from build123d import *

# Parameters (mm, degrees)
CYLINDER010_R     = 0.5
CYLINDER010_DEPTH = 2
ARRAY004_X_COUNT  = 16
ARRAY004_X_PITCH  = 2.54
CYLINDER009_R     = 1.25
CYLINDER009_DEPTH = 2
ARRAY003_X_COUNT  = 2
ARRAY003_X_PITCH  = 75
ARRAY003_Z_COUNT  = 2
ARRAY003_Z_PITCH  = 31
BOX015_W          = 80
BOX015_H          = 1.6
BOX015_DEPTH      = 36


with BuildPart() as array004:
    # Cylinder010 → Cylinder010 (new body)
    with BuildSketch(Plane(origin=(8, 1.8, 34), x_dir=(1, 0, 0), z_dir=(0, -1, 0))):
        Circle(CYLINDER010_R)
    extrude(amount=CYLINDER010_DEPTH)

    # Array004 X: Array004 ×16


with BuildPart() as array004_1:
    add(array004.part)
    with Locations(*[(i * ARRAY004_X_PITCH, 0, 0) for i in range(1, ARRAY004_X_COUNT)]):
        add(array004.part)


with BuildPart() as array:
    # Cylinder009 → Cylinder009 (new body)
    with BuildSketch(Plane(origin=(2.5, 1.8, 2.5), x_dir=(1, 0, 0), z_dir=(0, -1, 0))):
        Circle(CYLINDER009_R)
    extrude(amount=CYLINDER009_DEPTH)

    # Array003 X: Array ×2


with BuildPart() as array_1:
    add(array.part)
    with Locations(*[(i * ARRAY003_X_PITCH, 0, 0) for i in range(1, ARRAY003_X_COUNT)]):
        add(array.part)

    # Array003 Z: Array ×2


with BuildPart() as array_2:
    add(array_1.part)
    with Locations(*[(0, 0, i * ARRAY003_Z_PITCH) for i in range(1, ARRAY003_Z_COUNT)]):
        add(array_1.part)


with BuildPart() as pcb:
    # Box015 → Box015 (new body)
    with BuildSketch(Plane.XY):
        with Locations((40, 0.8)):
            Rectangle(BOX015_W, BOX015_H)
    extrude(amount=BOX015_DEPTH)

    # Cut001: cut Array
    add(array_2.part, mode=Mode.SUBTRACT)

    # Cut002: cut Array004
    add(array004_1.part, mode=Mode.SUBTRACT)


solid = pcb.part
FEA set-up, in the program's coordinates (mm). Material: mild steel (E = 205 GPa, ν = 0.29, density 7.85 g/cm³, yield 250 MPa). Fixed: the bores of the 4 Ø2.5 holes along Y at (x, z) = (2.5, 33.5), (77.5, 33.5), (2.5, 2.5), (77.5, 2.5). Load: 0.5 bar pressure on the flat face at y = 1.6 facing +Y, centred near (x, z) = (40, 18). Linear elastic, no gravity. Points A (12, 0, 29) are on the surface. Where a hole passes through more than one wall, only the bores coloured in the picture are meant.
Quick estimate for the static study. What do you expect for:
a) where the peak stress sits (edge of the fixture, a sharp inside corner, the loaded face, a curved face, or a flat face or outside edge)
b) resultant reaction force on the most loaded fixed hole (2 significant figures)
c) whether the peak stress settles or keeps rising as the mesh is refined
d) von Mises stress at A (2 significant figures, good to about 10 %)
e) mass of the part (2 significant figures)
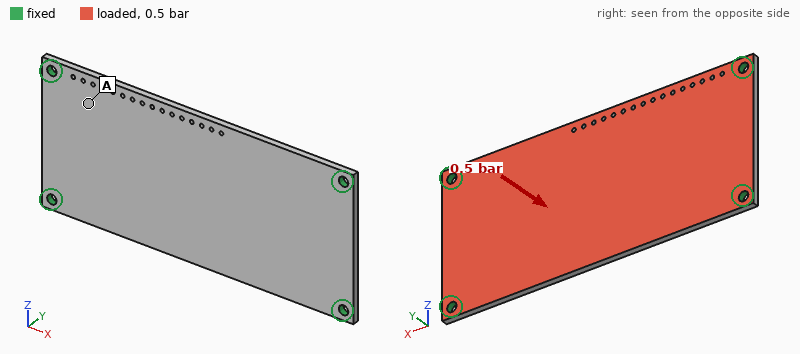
edge of the fixture
36 N
keeps rising
17 MPa
36 g
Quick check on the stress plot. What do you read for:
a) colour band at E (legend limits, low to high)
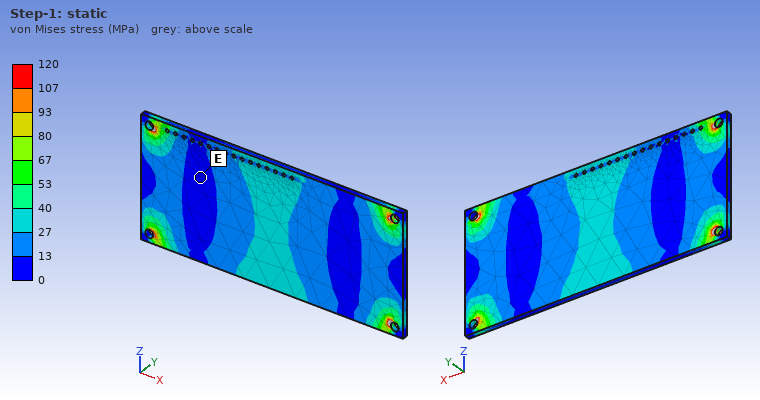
0 to 13 MPa
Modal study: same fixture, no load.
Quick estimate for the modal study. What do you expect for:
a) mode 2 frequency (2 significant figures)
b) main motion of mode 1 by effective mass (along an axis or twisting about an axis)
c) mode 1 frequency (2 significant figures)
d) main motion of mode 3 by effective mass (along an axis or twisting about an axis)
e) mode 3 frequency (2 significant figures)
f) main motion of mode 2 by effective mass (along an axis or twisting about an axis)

2600 Hz
along Y
1300 Hz
twisting about Z
3700 Hz
twisting about X
